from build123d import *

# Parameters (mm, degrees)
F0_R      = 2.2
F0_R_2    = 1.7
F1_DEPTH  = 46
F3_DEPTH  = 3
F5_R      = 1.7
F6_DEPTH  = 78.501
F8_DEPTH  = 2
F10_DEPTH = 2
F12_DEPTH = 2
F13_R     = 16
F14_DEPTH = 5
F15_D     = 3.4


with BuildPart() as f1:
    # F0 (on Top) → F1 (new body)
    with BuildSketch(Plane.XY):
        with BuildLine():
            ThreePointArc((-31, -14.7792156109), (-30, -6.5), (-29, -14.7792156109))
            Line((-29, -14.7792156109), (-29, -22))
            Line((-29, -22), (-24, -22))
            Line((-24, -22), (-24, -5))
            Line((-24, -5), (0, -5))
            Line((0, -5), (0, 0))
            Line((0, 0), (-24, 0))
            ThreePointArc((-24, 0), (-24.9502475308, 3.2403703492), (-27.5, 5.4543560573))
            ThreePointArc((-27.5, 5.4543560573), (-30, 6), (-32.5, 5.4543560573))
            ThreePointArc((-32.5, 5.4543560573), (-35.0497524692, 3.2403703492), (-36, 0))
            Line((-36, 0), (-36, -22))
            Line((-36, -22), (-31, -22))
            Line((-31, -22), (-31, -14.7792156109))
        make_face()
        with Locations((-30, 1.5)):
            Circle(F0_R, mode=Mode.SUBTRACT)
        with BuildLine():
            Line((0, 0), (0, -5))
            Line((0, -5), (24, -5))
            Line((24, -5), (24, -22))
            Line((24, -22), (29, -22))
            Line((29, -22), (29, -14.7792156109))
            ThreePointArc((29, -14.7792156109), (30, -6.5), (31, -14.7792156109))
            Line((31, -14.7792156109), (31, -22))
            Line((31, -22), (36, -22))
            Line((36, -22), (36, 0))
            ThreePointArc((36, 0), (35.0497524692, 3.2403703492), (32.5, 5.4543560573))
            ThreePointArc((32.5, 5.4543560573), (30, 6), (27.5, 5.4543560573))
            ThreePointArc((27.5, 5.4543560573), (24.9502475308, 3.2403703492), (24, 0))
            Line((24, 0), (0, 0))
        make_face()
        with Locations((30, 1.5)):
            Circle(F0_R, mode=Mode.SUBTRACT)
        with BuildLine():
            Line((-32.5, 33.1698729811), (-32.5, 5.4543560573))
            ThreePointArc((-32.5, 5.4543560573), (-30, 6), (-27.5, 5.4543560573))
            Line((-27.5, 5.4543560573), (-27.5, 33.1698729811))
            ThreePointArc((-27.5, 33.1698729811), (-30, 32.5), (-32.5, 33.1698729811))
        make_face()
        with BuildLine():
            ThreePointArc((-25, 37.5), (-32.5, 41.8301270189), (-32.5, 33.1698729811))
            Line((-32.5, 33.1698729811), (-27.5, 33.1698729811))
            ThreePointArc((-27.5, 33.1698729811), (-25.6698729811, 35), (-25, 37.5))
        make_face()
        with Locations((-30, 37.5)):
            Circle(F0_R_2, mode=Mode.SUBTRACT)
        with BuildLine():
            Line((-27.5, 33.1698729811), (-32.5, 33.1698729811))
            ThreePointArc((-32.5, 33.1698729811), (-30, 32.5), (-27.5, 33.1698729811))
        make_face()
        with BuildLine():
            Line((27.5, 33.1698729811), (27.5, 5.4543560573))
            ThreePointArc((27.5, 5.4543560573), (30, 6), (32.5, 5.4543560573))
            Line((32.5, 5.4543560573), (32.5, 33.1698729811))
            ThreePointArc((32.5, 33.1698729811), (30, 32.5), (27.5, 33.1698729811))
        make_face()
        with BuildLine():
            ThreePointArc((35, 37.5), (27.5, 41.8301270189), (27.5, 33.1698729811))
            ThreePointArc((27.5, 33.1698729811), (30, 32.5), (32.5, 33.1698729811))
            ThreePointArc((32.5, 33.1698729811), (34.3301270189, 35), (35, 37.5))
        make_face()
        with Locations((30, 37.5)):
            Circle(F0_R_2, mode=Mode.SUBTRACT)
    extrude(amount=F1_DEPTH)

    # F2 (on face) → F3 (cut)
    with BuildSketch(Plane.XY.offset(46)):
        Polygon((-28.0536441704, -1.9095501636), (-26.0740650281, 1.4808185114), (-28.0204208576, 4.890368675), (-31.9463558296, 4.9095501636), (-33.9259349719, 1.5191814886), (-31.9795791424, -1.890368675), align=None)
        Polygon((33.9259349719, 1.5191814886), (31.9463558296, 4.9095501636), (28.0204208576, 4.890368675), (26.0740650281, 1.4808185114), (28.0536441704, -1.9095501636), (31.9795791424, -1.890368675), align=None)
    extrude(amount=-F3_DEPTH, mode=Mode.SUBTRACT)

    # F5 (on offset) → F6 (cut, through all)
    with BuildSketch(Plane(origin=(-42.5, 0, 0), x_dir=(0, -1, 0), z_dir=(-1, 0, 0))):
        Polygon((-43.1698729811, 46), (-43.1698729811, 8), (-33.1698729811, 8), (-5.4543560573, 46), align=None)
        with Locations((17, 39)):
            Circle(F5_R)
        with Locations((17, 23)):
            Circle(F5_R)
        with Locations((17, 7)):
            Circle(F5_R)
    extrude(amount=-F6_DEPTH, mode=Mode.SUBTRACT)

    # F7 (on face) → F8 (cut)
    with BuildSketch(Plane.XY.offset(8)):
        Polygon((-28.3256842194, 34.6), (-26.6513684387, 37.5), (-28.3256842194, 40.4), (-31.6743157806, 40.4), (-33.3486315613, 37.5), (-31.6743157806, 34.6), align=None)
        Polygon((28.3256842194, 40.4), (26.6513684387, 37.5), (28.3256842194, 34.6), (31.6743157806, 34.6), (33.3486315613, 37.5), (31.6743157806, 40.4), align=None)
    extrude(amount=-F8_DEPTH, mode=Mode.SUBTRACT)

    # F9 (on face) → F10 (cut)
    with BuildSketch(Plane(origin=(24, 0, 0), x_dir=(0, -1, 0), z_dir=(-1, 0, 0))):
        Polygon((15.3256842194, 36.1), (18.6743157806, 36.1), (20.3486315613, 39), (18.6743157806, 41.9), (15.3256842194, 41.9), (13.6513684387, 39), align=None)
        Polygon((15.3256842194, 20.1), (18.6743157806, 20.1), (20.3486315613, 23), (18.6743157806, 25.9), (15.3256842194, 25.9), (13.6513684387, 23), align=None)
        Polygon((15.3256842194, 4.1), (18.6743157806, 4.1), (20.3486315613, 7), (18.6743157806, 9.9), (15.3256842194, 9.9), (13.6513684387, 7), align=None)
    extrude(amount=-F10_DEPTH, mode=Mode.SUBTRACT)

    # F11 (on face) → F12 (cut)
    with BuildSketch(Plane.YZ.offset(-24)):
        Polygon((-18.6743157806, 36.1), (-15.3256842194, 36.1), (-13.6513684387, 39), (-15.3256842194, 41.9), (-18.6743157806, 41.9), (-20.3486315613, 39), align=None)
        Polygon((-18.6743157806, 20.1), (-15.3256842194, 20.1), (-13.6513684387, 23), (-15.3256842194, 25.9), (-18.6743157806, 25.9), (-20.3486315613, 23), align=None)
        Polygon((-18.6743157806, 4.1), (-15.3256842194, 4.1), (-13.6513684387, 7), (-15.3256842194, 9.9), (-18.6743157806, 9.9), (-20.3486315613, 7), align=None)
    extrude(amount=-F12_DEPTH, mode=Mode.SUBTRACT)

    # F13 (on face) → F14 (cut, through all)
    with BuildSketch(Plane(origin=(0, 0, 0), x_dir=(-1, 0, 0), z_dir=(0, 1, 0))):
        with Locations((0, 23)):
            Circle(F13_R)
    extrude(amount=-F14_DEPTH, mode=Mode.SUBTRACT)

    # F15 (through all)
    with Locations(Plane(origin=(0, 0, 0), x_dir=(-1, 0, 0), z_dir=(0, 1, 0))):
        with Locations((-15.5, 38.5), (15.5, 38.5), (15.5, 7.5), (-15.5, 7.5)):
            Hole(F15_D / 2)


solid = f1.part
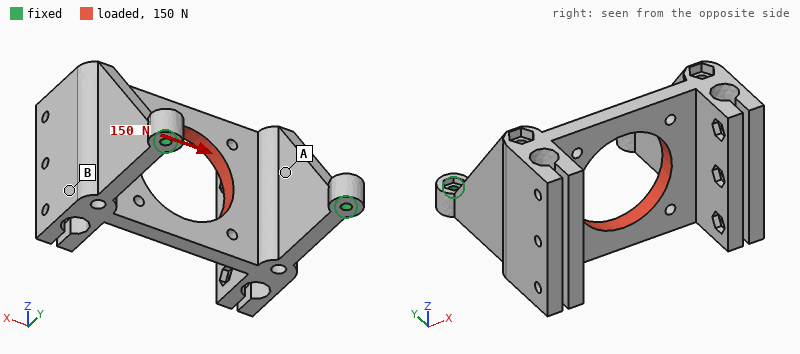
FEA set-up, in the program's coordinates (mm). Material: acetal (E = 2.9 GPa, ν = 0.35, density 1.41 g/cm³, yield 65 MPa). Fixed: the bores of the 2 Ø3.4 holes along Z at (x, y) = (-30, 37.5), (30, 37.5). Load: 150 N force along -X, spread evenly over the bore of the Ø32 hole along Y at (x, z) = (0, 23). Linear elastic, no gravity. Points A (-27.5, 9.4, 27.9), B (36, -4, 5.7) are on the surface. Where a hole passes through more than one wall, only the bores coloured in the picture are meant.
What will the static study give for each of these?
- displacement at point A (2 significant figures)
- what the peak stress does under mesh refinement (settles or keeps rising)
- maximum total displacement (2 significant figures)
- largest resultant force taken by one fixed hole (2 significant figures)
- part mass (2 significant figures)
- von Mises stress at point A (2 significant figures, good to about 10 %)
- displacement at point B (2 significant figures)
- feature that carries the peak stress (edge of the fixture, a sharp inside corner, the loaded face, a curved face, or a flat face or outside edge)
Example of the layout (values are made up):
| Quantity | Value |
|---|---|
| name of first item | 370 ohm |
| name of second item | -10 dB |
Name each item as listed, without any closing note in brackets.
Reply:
| Quantity | Value |
|---|---|
| displacement at point A | 0.77 mm |
| what the peak stress does under mesh refinement | keeps rising |
| maximum total displacement | 1.2 mm |
| largest resultant force taken by one fixed hole | 100 N |
| part mass | 51 g |
| von Mises stress at point A | 5.4 MPa |
| displacement at point B | 0.86 mm |
| feature that carries the peak stress | edge of the fixture |
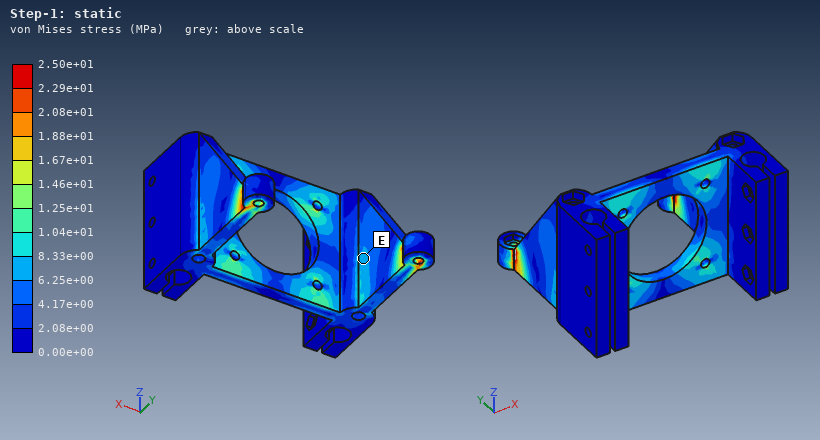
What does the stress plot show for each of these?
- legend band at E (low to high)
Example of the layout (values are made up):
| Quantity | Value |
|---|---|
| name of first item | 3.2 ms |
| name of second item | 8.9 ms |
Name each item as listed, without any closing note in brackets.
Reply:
| Quantity | Value |
|---|---|
| legend band at E | 6.25e+00 to 8.33e+00 MPa |
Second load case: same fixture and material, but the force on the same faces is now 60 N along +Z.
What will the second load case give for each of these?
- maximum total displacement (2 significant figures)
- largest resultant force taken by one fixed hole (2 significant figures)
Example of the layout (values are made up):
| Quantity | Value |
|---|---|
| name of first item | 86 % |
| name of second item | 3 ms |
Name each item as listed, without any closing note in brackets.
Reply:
| Quantity | Value |
|---|---|
| maximum total displacement | 1.2 mm |
| largest resultant force taken by one fixed hole | 30 N |
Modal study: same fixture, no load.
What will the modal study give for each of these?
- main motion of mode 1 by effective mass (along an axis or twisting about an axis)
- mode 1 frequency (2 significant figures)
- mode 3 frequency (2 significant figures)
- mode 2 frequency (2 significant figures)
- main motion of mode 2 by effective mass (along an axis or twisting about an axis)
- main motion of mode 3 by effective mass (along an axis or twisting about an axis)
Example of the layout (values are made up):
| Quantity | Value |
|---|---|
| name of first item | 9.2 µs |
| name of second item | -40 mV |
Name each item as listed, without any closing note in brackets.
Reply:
| Quantity | Value |
|---|---|
| main motion of mode 1 by effective mass | along Z |
| mode 1 frequency | 180 Hz |
| mode 3 frequency | 300 Hz |
| mode 2 frequency | 290 Hz |
| main motion of mode 2 by effective mass | along X |
| main motion of mode 3 by effective mass | along X |
